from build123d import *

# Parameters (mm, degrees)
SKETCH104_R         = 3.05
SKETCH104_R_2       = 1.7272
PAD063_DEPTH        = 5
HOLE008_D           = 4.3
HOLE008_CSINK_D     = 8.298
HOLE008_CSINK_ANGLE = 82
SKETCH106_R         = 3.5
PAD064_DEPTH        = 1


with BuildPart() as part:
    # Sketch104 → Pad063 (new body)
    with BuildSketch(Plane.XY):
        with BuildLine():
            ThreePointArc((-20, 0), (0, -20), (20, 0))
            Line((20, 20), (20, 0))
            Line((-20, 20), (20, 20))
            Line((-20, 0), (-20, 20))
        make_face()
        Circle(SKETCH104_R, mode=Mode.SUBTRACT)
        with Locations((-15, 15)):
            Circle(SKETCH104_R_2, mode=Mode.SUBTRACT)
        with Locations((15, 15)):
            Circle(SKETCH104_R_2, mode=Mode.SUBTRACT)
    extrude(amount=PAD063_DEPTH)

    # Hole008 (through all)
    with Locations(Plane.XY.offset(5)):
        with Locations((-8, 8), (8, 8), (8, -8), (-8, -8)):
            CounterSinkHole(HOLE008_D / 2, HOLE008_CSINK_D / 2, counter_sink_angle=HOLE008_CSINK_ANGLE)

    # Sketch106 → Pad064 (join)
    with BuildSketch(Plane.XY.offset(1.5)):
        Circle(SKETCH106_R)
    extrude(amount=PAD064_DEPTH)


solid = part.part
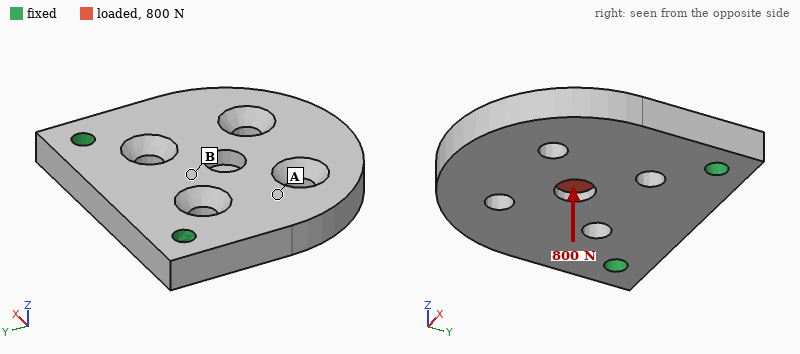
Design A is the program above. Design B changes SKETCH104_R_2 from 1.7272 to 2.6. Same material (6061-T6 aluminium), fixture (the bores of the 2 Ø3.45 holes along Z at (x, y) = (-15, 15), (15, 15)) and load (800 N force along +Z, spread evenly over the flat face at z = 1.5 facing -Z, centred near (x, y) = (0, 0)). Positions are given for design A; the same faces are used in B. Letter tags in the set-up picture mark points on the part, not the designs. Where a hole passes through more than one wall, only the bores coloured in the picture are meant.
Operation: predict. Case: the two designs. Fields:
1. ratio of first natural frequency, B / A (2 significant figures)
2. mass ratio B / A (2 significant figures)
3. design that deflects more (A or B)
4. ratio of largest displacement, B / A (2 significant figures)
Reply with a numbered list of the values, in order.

1. 1.1
2. 0.98
3. A
4. 0.83
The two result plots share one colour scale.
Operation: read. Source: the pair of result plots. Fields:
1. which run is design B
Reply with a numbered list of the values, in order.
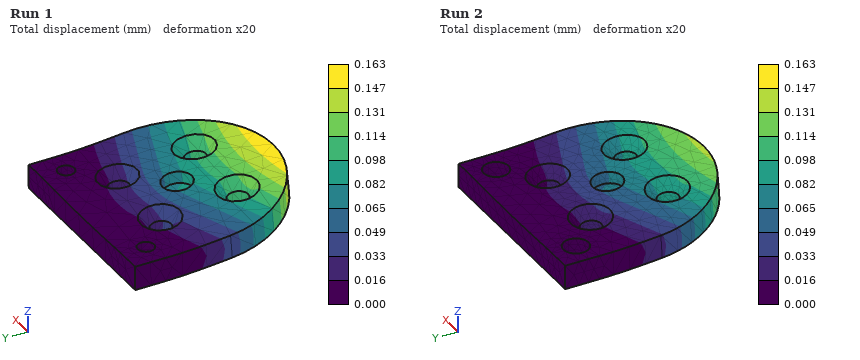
1. Run 2
